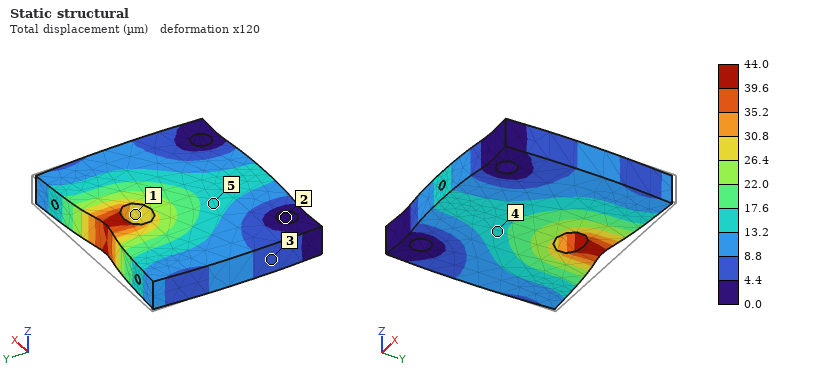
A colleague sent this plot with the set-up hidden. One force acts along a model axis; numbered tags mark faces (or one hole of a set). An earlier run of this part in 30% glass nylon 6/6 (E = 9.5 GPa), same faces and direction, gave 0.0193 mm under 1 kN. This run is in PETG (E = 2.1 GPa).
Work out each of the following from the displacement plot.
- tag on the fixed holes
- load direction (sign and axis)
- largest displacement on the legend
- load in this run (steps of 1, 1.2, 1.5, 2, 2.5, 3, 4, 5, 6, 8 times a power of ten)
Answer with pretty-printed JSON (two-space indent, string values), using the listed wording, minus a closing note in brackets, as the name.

{
  "tag on the fixed holes": "2",
  "load direction": "-Y",
  "largest displacement on the legend": "44.0 µm",
  "load in this run": "500 N"
}
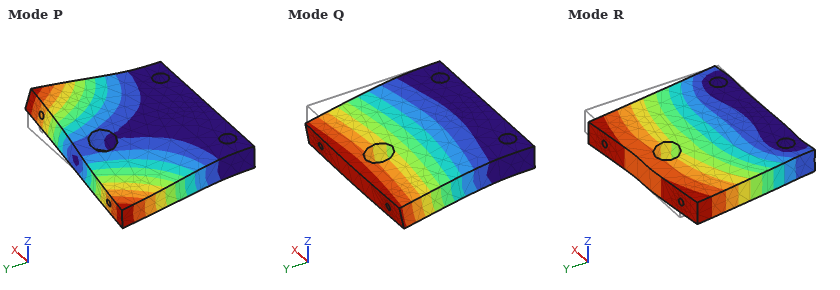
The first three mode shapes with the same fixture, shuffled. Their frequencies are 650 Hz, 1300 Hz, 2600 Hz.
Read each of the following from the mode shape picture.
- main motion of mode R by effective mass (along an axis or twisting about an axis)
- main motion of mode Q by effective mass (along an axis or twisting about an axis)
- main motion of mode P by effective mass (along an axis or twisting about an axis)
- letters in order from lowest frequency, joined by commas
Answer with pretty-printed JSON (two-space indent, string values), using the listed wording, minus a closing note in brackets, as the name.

{
  "main motion of mode R by effective mass": "along X",
  "main motion of mode Q by effective mass": "along Z",
  "main motion of mode P by effective mass": "twisting about Y",
  "letters in order from lowest frequency, joined by commas": "Q, P, R"
}
